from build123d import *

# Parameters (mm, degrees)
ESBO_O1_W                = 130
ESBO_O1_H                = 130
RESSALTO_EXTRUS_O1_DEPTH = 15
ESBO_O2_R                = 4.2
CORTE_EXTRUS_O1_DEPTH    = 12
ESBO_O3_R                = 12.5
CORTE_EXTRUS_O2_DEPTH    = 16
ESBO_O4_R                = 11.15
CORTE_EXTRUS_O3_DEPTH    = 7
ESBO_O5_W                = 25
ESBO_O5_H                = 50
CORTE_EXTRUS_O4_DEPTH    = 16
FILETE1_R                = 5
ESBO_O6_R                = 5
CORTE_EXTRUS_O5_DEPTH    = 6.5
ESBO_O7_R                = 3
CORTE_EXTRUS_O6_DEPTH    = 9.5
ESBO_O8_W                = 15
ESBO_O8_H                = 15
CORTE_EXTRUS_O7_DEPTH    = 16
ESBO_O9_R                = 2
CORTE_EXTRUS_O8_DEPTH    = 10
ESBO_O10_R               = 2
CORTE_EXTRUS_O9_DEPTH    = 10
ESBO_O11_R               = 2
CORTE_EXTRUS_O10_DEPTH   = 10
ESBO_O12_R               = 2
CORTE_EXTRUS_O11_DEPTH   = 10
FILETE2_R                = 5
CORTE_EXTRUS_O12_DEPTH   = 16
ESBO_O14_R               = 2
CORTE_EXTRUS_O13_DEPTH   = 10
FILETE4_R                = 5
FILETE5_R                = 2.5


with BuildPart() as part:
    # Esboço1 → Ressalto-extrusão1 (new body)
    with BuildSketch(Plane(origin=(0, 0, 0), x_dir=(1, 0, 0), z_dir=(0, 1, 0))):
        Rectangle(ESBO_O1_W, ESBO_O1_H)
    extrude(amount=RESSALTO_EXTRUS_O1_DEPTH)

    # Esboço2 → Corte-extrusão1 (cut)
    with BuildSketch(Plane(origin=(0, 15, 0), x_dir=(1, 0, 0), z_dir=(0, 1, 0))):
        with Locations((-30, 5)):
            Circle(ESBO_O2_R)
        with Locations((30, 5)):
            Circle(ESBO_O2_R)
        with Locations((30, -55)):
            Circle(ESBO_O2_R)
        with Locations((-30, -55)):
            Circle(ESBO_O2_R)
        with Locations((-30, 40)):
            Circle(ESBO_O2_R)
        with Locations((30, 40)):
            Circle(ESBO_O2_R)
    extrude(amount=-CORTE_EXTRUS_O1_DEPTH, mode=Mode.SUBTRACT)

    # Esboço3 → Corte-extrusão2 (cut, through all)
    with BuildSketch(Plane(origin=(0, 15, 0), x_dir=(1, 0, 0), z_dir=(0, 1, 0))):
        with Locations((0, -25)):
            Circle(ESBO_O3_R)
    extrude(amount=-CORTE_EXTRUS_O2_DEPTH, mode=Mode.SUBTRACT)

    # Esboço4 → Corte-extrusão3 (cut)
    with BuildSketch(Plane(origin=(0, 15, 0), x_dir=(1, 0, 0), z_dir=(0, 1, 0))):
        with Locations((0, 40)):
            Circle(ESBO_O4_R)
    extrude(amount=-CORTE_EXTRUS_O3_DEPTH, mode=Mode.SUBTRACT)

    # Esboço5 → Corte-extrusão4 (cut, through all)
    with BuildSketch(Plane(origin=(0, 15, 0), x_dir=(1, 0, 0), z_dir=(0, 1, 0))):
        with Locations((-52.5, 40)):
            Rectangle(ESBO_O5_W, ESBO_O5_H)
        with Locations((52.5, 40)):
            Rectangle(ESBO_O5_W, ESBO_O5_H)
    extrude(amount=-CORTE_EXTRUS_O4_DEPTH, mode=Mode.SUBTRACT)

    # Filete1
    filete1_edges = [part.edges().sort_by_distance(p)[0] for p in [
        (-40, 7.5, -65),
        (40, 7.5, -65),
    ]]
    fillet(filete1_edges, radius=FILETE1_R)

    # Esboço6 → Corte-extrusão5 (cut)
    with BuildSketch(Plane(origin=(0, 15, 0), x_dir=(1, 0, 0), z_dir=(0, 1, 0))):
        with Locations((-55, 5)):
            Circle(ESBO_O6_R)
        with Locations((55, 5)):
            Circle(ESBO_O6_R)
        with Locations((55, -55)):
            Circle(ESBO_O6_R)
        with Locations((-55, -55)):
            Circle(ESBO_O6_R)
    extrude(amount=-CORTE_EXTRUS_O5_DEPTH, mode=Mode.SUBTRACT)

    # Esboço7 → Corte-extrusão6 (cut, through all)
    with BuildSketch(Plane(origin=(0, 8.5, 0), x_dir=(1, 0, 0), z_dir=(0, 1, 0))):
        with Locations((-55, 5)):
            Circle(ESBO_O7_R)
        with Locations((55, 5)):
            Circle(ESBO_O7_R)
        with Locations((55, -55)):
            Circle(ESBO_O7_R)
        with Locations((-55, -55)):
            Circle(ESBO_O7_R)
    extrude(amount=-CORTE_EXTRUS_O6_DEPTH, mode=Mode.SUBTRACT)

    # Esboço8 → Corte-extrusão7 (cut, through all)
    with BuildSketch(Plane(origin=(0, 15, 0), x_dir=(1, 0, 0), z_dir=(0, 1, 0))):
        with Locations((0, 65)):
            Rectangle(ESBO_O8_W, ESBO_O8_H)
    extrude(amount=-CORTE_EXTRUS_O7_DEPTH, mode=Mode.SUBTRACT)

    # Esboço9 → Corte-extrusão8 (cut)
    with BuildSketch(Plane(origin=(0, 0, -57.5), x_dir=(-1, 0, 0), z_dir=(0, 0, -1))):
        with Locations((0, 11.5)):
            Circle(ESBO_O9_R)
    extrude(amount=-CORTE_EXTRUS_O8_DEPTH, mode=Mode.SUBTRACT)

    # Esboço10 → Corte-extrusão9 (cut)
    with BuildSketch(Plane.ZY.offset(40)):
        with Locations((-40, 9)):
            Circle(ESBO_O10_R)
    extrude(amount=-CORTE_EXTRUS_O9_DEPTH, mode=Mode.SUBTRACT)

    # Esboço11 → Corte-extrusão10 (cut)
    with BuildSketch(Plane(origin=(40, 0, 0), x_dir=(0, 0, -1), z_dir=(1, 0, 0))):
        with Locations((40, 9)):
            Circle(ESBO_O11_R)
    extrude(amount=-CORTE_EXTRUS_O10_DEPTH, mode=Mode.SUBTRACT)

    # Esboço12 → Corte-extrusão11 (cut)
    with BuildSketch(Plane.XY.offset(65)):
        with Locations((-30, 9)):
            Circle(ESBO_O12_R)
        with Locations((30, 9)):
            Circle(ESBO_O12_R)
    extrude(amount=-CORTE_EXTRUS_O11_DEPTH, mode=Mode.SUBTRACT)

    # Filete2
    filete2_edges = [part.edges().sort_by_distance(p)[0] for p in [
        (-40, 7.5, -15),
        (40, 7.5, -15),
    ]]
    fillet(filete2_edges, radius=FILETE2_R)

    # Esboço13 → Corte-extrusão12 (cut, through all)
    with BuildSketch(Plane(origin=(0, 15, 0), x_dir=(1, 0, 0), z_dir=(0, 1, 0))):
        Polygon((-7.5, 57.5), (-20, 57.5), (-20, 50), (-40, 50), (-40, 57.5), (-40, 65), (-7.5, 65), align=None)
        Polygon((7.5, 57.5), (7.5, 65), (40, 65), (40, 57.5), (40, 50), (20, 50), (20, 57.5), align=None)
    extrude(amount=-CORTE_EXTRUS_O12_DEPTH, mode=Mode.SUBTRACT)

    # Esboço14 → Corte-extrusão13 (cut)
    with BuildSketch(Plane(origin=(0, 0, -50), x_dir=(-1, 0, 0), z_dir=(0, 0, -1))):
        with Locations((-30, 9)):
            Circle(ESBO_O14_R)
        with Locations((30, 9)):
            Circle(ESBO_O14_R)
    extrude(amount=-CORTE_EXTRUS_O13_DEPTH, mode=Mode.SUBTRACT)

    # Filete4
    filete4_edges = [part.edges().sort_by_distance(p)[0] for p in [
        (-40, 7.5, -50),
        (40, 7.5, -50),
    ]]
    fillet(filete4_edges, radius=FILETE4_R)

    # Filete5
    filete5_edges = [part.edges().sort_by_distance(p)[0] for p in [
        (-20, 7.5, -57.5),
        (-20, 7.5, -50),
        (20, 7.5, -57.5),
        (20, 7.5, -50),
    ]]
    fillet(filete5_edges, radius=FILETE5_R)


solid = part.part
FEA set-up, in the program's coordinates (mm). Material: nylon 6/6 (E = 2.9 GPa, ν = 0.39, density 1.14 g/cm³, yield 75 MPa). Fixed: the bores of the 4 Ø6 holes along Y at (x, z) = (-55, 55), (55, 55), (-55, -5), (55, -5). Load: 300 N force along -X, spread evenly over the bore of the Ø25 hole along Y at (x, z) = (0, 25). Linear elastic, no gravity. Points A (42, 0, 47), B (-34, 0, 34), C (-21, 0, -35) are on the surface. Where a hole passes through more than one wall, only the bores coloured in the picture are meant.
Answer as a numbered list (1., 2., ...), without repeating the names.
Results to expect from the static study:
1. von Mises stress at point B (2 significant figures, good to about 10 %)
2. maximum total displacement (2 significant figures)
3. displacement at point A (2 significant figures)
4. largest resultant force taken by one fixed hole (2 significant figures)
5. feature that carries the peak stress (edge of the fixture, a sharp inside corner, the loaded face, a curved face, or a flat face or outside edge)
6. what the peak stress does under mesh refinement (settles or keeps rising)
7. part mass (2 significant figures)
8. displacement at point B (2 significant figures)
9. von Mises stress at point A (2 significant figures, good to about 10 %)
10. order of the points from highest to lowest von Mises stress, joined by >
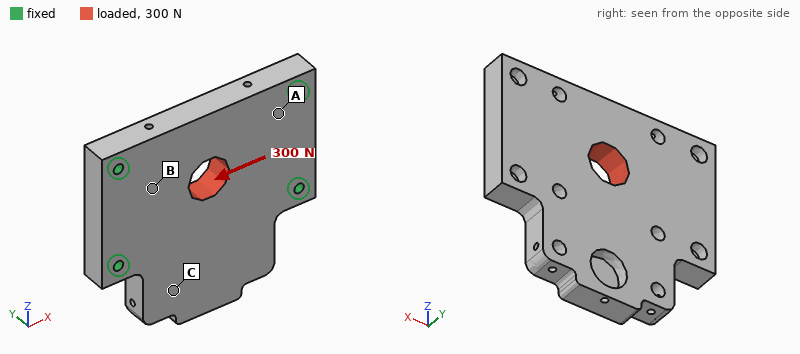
1. 0.18 MPa
2. 5.2 µm
3. 1.9 µm
4. 78 N
5. edge of the fixture
6. keeps rising
7. 210 g
8. 3.2 µm
9. 0.32 MPa
10. A > B > C
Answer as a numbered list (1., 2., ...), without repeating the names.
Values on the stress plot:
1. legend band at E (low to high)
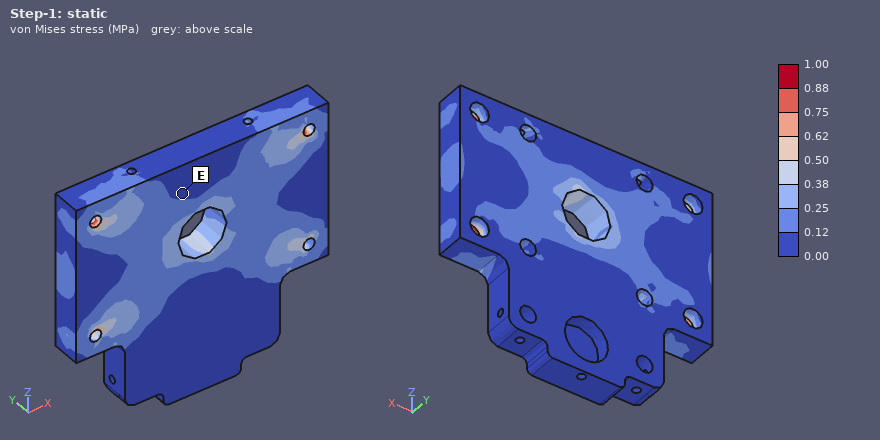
1. 0.00 to 0.12 MPa
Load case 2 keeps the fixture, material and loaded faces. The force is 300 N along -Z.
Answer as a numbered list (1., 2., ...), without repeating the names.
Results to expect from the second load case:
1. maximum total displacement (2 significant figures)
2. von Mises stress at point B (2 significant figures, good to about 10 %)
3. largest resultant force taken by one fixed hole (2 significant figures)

1. 9.5 µm
2. 0.27 MPa
3. 89 N
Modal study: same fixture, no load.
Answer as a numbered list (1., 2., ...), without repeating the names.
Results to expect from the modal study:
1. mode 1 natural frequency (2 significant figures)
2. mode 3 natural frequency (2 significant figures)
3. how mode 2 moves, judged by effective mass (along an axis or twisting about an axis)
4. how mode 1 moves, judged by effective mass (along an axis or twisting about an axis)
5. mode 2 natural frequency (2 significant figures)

1. 770 Hz
2. 2000 Hz
3. along Y
4. along Y
5. 1400 Hz
